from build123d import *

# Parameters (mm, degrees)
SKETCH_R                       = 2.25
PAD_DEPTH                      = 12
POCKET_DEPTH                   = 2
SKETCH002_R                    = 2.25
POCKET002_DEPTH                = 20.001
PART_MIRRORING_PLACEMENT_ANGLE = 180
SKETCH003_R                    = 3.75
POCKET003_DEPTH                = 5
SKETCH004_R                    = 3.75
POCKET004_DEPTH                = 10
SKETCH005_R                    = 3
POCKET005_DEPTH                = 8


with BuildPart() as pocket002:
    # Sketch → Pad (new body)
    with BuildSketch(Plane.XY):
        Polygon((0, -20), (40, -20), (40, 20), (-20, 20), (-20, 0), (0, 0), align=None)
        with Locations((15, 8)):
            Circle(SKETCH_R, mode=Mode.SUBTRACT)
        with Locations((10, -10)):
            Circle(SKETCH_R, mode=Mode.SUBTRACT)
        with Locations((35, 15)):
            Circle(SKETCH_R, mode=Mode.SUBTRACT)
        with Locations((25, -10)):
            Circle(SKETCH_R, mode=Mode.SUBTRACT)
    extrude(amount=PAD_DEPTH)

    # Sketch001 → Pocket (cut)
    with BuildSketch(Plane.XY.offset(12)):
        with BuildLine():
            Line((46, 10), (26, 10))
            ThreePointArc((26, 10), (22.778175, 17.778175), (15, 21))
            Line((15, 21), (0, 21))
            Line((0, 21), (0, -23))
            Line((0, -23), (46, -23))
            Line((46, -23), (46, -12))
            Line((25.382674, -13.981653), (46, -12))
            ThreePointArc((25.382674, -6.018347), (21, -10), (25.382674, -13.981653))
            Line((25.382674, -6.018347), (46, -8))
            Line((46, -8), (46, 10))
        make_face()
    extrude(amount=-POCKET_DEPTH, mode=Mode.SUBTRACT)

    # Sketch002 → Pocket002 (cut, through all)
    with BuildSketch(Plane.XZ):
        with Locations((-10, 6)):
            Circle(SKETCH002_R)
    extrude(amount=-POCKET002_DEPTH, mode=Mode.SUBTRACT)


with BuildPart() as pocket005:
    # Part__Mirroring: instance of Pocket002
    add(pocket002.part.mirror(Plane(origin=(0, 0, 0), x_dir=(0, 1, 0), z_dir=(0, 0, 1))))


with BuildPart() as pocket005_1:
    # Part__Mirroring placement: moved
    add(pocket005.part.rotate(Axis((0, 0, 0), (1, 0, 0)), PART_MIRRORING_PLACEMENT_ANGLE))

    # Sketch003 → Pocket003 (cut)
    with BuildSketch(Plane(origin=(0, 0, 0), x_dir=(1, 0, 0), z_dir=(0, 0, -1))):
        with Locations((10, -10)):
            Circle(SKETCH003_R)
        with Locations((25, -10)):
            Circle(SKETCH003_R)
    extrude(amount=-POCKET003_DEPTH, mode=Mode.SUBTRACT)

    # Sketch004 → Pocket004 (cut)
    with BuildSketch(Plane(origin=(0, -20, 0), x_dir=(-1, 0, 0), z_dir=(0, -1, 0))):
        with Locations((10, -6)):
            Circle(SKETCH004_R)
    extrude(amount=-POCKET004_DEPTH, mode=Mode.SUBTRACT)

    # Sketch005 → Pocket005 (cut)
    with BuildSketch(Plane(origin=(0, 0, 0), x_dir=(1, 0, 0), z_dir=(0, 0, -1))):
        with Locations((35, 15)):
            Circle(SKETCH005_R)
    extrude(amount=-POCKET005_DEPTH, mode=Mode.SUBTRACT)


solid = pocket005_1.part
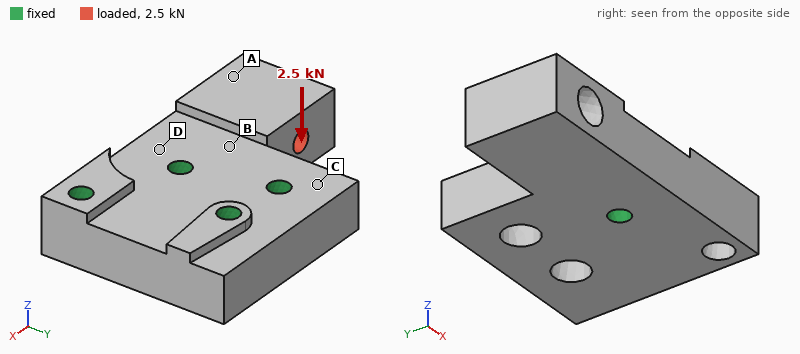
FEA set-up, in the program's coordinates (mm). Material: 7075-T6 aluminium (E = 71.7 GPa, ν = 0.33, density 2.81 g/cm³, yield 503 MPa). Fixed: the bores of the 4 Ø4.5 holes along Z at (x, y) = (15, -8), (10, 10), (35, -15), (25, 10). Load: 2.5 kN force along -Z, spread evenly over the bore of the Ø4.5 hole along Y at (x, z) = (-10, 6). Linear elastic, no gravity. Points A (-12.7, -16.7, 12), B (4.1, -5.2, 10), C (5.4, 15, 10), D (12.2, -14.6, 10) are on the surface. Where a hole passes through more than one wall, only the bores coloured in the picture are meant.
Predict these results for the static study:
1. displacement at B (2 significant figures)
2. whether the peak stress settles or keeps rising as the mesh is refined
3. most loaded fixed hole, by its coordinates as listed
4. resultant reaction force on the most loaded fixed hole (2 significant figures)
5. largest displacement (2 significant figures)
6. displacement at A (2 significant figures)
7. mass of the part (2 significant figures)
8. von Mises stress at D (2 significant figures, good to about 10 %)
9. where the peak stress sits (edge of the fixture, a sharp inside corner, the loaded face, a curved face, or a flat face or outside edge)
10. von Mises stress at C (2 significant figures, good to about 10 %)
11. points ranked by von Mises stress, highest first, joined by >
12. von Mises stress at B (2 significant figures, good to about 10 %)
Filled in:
0.030 mm
keeps rising
(15, -8)
2.5 kN
0.16 mm
0.11 mm
55 g
77 MPa
edge of the fixture
26 MPa
B > D > C > A
100 MPa
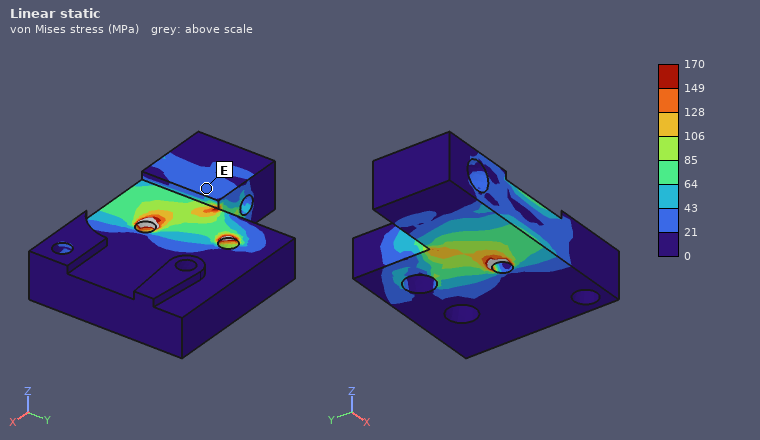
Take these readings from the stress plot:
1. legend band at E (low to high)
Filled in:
21 to 43 MPa
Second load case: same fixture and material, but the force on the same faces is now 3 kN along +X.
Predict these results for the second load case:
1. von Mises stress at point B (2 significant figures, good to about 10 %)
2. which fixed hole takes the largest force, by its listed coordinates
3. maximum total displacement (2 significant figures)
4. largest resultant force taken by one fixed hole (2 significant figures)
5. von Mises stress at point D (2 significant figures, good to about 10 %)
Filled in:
31 MPa
(15, -8)
16 µm
2.2 kN
10 MPa
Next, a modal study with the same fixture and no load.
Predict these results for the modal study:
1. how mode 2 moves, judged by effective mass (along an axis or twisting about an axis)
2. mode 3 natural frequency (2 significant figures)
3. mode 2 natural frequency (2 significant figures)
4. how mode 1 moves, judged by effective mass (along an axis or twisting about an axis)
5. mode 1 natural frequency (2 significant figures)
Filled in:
along Y
19 kHz
13 kHz
along Z
6600 Hz
